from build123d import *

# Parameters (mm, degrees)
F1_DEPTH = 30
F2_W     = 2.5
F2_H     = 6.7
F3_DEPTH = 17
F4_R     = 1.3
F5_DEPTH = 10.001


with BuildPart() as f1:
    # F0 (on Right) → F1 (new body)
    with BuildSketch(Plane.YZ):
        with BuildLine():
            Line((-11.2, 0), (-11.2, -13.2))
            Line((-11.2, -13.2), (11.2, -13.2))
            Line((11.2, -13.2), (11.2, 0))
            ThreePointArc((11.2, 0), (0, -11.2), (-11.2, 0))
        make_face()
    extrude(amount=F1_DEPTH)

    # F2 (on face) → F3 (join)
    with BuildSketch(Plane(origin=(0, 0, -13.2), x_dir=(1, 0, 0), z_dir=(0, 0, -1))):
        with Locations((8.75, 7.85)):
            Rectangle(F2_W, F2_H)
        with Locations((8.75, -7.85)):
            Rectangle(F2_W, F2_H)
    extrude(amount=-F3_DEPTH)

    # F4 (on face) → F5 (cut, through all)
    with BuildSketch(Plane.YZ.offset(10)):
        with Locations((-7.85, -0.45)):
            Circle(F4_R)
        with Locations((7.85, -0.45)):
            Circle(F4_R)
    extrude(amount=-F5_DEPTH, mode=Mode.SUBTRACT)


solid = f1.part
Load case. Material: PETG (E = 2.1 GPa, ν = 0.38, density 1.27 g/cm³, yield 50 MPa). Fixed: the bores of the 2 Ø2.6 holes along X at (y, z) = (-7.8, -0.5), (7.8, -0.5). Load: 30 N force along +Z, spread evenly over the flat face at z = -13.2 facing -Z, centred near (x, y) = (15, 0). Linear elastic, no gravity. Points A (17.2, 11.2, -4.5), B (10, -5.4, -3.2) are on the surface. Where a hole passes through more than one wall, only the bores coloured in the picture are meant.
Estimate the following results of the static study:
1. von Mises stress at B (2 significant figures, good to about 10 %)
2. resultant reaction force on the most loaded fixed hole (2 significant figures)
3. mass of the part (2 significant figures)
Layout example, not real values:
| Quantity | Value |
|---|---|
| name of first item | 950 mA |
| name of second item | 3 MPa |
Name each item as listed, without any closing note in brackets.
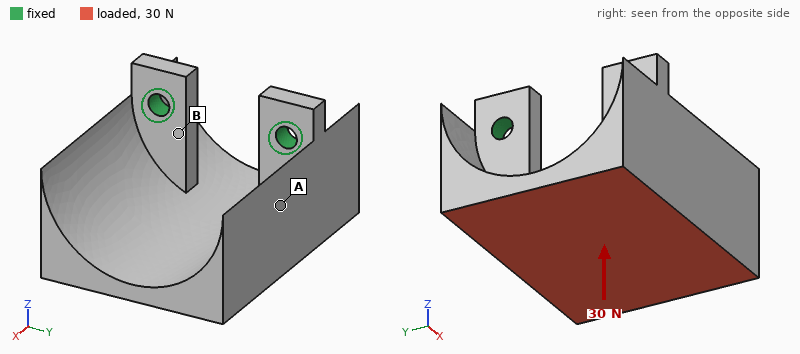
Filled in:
| Quantity | Value |
|---|---|
| von Mises stress at B | 8.5 MPa |
| resultant reaction force on the most loaded fixed hole | 15 N |
| mass of the part | 4.2 g |
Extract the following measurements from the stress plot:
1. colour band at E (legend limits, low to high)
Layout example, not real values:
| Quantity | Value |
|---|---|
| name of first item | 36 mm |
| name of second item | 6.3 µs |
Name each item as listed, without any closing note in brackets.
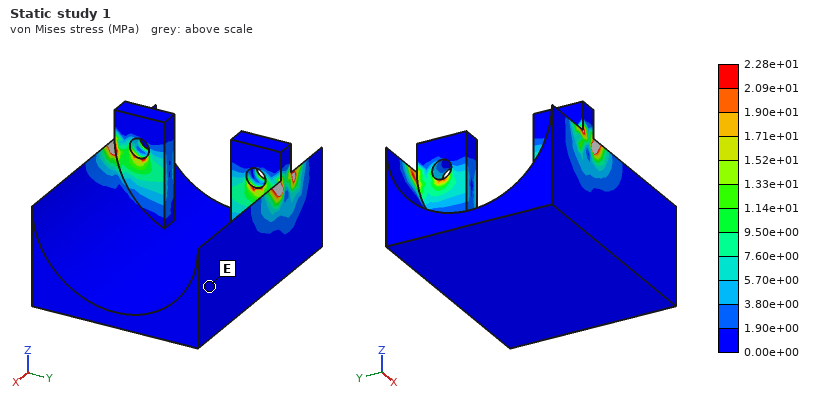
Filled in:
| Quantity | Value |
|---|---|
| colour band at E | 0.00e+00 to 1.90e+00 MPa |
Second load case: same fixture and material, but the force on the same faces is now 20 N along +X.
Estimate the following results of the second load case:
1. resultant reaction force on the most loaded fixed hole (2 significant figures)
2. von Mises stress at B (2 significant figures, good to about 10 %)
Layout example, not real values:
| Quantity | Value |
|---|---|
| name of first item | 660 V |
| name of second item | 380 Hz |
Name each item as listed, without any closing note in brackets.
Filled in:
| Quantity | Value |
|---|---|
| resultant reaction force on the most loaded fixed hole | 10 N |
| von Mises stress at B | 9.1 MPa |
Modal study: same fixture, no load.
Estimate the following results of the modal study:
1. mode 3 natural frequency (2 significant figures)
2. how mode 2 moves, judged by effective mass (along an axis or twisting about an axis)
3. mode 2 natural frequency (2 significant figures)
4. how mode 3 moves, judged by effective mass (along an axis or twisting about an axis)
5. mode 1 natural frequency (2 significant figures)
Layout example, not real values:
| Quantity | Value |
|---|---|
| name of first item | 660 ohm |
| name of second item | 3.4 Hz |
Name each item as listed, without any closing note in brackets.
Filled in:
| Quantity | Value |
|---|---|
| mode 3 natural frequency | 2600 Hz |
| how mode 2 moves, judged by effective mass | along Y |
| mode 2 natural frequency | 1400 Hz |
| how mode 3 moves, judged by effective mass | along Y |
| mode 1 natural frequency | 640 Hz |
